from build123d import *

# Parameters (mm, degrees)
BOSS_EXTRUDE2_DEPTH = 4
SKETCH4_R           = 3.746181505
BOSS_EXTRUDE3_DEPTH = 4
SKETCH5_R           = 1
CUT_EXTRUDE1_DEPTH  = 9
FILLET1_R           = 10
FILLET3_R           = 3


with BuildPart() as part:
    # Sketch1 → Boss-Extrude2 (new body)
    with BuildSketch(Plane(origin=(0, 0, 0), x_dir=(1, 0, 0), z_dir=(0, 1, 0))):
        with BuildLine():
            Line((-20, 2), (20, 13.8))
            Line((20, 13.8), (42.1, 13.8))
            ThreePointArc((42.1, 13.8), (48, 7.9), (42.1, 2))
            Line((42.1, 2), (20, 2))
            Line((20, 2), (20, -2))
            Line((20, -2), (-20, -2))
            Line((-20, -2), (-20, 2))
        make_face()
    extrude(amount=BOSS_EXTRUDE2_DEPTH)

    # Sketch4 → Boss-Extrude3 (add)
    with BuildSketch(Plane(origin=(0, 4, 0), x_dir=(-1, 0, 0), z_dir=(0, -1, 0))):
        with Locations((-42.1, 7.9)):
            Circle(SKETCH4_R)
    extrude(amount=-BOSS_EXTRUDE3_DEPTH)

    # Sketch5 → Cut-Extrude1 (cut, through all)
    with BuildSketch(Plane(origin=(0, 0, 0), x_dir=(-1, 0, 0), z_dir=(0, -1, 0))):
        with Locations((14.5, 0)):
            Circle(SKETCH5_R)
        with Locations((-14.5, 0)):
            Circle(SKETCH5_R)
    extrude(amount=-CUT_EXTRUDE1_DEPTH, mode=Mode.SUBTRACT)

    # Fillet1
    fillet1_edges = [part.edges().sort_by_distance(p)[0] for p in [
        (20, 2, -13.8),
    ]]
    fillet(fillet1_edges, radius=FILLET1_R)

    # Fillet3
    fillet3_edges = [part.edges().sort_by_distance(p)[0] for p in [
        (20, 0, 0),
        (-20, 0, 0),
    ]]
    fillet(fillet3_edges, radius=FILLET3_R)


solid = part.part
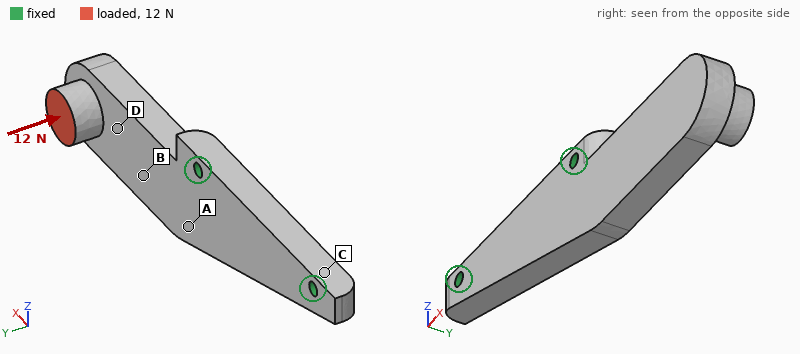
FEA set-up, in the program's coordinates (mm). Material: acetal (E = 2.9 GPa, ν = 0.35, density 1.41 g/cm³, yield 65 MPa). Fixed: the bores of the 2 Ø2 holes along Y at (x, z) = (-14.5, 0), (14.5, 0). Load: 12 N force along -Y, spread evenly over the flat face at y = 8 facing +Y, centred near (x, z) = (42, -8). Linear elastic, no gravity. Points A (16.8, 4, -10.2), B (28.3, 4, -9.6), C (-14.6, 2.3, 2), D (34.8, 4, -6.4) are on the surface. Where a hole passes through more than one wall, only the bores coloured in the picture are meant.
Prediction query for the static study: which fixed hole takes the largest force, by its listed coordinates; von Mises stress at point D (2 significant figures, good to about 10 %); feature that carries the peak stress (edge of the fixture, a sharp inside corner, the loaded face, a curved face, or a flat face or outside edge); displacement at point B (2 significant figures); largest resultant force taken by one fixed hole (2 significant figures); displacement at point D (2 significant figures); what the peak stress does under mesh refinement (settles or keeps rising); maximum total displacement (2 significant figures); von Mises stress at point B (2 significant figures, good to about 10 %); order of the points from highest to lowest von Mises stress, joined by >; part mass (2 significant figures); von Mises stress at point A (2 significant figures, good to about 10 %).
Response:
(14.5, 0)
2.9 MPa
edge of the fixture
0.25 mm
17 N
0.41 mm
keeps rising
0.81 mm
5.2 MPa
A > B > D > C
4.2 g
7.3 MPa
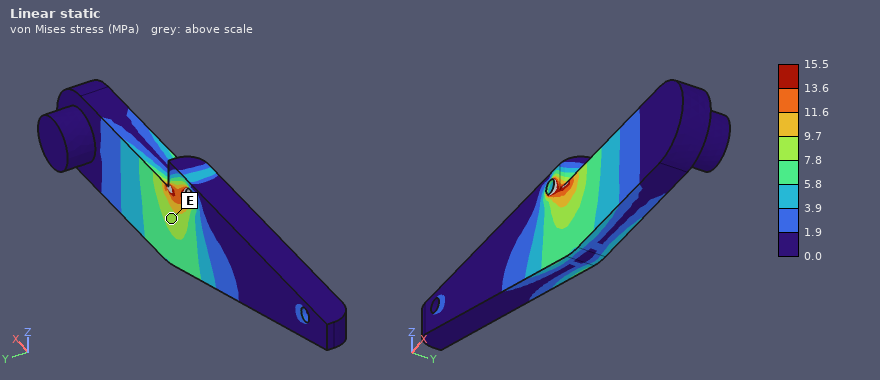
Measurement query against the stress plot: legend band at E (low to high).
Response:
7.8 to 9.7 MPa
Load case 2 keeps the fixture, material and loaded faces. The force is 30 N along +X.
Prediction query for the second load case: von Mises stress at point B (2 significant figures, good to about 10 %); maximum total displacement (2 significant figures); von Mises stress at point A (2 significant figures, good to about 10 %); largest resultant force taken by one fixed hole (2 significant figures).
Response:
6.3 MPa
0.63 mm
5.4 MPa
17 N
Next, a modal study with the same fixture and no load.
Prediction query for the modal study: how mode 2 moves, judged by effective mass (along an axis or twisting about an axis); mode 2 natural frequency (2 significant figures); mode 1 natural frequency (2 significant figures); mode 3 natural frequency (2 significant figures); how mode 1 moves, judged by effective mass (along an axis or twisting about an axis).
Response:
along Z
1600 Hz
650 Hz
2600 Hz
along Y
